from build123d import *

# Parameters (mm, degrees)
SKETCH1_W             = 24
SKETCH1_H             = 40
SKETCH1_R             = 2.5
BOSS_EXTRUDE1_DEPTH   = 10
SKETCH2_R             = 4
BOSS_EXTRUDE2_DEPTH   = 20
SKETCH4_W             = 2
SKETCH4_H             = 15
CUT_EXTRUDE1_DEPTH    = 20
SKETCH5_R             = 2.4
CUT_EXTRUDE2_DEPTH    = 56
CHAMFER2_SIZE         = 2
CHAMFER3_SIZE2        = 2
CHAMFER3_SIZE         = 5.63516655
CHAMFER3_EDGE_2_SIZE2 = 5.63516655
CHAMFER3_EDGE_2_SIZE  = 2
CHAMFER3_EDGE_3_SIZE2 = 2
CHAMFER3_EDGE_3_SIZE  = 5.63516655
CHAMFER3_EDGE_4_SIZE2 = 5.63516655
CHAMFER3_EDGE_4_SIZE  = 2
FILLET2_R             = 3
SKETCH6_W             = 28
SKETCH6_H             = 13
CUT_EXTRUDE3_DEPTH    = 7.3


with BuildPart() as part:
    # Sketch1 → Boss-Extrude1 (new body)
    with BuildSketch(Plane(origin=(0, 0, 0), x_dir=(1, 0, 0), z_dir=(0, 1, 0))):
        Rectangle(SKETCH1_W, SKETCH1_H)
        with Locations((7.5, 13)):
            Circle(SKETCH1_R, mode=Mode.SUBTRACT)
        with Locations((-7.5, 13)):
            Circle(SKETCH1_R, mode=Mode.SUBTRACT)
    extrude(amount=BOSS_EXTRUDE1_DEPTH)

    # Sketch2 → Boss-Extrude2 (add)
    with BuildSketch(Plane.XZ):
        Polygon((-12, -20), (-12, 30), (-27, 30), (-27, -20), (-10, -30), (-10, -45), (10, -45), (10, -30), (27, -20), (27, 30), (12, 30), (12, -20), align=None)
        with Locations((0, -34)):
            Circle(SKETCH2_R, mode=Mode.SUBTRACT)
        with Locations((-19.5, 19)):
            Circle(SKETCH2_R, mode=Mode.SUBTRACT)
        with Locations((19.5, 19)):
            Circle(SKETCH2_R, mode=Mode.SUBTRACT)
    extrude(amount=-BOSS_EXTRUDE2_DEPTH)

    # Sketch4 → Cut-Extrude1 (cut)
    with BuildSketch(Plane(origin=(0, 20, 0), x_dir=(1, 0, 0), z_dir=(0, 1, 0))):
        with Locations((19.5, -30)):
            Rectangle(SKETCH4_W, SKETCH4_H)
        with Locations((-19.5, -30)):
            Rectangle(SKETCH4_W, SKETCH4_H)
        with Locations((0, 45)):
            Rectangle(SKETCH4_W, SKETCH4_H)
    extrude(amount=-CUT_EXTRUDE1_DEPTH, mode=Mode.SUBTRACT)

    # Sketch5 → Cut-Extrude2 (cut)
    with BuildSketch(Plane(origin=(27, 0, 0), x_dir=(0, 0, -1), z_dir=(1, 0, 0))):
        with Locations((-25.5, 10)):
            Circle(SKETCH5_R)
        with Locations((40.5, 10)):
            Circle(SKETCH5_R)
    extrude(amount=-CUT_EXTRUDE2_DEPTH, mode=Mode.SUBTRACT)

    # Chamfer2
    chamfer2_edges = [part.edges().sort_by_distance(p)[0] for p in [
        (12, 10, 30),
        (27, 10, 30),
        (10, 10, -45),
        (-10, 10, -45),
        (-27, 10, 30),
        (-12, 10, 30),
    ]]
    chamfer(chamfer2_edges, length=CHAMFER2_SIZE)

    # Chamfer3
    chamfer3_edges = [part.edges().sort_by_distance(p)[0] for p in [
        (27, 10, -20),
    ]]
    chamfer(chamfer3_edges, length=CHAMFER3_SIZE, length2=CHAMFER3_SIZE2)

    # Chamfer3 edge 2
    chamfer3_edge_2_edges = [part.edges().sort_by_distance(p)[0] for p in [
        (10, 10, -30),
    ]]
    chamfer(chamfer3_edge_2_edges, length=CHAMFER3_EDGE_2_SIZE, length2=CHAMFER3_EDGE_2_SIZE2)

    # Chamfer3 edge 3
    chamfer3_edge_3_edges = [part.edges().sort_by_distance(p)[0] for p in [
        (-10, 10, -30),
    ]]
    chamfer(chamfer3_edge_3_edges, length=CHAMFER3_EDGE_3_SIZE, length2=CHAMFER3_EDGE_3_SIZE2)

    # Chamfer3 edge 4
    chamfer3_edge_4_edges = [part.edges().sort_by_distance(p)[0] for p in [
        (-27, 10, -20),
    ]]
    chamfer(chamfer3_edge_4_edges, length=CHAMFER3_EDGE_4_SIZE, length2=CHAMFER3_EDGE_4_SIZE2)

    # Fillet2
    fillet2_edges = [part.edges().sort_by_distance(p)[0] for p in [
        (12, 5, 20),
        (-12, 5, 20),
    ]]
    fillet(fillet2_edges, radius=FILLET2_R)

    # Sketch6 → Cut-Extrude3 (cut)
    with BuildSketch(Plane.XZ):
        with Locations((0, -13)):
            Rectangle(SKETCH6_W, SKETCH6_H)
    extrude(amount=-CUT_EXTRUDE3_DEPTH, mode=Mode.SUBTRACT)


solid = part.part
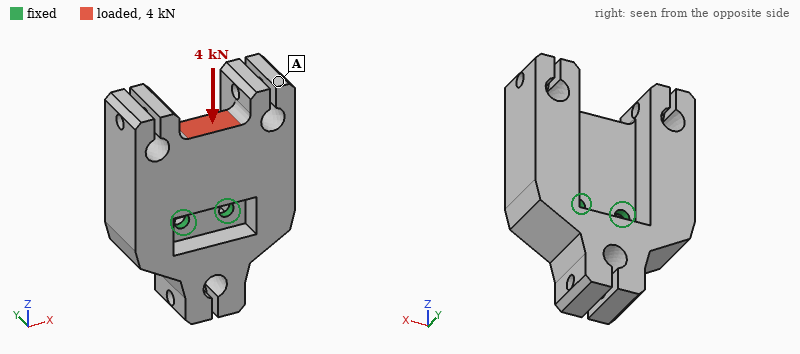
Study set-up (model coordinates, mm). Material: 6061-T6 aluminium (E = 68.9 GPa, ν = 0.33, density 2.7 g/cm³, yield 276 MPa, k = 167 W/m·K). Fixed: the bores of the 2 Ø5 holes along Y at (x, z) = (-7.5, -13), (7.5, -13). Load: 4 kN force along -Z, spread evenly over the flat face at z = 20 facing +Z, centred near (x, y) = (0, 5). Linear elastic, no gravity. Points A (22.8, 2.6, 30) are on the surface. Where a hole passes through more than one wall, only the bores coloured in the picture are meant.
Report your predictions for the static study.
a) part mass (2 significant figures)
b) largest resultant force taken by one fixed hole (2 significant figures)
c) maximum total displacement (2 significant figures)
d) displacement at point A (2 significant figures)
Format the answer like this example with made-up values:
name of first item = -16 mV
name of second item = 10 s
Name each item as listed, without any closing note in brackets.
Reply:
part mass = 120 g
largest resultant force taken by one fixed hole = 2.0 kN
maximum total displacement = 0.17 mm
displacement at point A = 0.17 mm
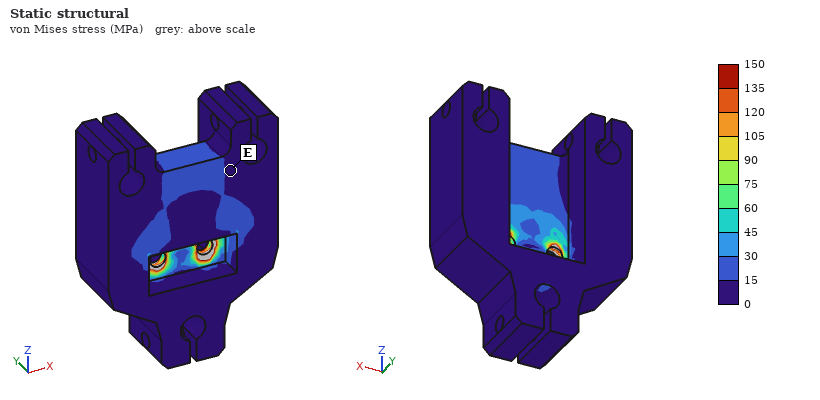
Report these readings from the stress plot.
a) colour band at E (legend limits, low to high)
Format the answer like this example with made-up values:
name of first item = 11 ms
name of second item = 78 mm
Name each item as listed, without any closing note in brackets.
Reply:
colour band at E = 0 to 15 MPa
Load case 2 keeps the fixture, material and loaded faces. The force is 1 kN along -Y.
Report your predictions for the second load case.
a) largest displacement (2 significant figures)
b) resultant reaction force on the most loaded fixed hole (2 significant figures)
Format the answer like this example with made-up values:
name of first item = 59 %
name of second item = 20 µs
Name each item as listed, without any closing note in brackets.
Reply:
largest displacement = 0.37 mm
resultant reaction force on the most loaded fixed hole = 500 N
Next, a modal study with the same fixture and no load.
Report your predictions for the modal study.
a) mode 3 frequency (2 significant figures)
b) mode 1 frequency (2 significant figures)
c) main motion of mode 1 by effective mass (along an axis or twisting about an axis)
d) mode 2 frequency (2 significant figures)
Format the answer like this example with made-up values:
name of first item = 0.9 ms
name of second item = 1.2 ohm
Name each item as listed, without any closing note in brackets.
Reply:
mode 3 frequency = 4300 Hz
mode 1 frequency = 1400 Hz
main motion of mode 1 by effective mass = along Y
mode 2 frequency = 3700 Hz
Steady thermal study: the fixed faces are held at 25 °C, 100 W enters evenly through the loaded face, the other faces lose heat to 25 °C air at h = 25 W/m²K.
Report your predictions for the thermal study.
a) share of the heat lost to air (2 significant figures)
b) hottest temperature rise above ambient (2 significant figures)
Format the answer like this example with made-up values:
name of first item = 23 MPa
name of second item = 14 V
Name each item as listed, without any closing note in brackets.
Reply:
share of the heat lost to air = 10 %
hottest temperature rise above ambient = 68 K
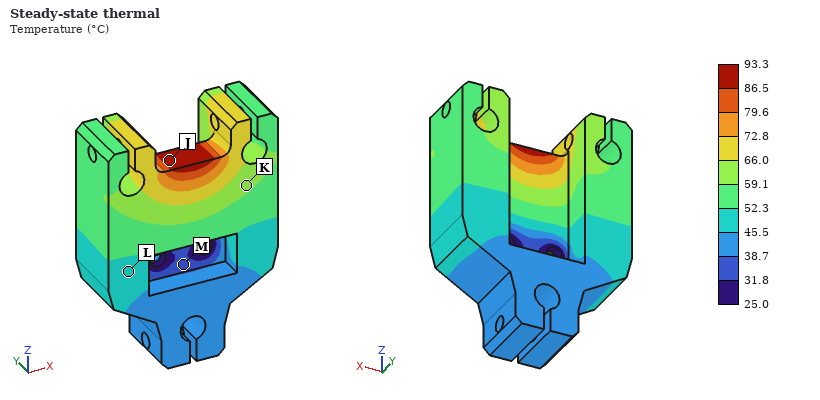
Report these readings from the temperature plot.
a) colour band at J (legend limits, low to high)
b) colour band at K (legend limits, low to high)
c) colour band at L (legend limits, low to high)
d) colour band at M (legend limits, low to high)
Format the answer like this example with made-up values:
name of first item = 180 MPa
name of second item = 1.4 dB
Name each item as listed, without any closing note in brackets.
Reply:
colour band at J = 86.5 to 93.3 °C
colour band at K = 59.1 to 66.0 °C
colour band at L = 45.5 to 52.3 °C
colour band at M = 31.8 to 38.7 °C
